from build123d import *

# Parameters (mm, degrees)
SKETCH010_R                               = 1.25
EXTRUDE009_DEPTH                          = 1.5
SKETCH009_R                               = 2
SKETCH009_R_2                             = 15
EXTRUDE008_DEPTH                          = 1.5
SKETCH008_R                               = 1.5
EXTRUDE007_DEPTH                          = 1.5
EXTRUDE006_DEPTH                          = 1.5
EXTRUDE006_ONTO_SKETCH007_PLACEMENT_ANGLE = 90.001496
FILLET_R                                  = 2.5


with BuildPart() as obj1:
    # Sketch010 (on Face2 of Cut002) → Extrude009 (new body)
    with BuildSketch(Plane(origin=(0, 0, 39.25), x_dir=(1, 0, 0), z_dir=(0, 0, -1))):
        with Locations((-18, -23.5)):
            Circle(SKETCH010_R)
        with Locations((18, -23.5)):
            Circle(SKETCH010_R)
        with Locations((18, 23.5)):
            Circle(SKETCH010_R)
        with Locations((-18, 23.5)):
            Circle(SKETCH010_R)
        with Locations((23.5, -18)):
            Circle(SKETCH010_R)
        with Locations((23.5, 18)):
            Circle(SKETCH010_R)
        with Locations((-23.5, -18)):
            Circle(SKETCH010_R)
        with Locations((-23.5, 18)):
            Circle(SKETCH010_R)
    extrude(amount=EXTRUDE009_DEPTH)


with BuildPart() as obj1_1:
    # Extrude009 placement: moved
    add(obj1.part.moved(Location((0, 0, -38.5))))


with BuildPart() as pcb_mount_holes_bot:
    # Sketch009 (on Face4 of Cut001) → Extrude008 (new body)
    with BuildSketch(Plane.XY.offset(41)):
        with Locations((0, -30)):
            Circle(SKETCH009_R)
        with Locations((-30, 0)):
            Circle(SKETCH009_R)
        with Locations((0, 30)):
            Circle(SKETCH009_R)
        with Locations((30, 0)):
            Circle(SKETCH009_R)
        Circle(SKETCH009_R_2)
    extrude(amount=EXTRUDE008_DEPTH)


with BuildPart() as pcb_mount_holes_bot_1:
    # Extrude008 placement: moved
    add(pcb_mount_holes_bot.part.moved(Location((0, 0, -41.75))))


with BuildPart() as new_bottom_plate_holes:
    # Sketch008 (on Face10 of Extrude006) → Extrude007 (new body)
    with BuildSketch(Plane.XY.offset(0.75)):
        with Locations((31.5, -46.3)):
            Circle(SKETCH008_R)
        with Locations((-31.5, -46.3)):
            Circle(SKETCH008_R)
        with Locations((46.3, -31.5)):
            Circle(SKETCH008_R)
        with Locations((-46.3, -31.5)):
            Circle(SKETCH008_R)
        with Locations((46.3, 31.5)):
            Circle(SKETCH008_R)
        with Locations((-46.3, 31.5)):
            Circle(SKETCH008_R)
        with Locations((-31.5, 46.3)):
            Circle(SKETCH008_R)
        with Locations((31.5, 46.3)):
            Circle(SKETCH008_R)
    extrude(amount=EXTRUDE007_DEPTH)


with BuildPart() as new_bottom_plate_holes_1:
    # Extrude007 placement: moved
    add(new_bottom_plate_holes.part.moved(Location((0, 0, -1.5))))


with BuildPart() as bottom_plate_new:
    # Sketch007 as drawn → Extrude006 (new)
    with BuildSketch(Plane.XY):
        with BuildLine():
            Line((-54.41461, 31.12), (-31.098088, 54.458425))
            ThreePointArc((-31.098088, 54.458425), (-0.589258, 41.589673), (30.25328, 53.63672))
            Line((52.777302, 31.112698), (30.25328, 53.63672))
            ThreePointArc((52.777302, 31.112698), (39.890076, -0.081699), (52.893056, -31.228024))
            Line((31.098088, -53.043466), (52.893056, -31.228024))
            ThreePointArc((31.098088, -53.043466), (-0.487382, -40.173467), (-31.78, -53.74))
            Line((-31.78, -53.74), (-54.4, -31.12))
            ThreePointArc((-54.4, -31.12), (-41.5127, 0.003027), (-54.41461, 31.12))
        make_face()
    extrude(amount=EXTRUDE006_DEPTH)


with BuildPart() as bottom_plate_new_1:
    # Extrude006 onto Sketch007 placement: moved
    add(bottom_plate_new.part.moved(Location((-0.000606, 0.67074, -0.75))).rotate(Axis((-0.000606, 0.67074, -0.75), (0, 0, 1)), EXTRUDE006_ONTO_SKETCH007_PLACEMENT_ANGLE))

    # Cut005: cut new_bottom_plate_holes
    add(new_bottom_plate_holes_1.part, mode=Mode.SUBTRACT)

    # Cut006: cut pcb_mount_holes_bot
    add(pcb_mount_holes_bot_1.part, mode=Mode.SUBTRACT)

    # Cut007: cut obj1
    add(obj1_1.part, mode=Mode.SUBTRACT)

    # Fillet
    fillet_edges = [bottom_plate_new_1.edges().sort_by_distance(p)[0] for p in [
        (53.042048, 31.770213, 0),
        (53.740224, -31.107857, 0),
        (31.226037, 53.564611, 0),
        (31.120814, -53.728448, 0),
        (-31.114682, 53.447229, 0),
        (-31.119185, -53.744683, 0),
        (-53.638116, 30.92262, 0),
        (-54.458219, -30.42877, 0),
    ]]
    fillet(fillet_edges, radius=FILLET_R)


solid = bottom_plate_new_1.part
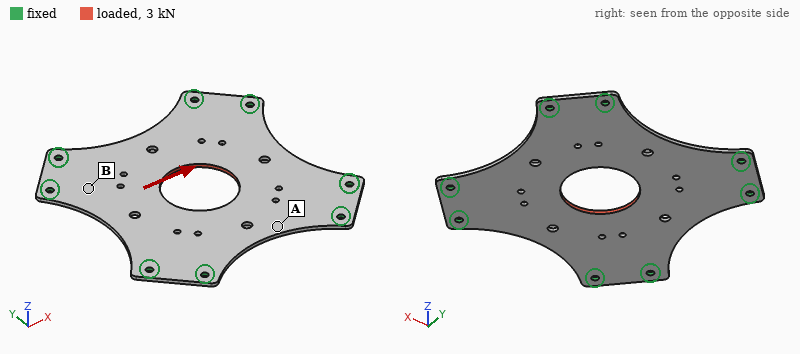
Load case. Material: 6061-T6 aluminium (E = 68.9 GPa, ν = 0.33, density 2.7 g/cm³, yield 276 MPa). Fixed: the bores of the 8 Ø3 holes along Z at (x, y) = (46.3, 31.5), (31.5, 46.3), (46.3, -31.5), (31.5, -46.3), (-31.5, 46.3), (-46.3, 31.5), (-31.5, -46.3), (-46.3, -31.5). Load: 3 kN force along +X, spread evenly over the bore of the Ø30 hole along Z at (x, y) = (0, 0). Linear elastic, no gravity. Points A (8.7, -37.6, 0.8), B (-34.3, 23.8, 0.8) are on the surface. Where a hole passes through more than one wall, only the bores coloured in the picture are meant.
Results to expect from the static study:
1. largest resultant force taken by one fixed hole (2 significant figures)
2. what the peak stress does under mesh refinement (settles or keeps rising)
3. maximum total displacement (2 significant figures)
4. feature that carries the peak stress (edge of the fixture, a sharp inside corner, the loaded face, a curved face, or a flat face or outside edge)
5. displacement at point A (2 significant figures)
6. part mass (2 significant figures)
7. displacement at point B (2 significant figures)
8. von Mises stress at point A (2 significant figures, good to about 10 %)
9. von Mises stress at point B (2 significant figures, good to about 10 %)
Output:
600 N
keeps rising
19 µm
edge of the fixture
5.6 µm
30 g
6.9 µm
9.0 MPa
22 MPa
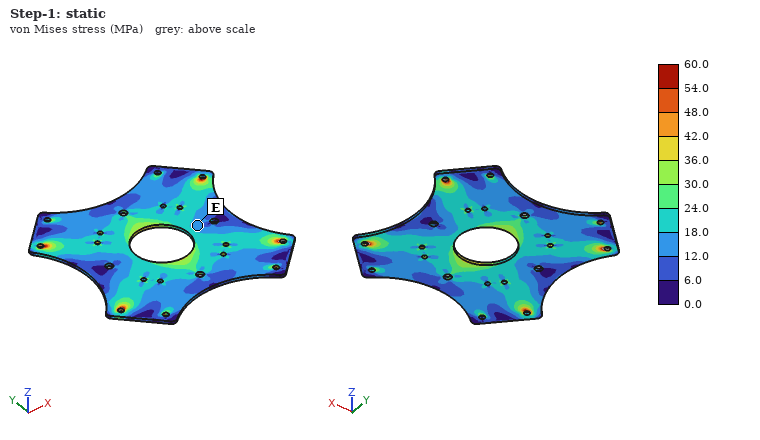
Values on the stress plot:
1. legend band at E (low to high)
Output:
12.0 to 18.0 MPa
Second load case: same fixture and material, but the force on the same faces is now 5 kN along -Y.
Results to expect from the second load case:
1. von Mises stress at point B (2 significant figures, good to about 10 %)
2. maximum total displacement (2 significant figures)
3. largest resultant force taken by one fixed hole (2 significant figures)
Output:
22 MPa
31 µm
1.0 kN
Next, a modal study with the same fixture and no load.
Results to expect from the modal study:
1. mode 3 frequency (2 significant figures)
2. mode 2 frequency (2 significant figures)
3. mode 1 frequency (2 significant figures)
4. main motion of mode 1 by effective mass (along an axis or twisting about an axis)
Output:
1800 Hz
1800 Hz
960 Hz
along Z
